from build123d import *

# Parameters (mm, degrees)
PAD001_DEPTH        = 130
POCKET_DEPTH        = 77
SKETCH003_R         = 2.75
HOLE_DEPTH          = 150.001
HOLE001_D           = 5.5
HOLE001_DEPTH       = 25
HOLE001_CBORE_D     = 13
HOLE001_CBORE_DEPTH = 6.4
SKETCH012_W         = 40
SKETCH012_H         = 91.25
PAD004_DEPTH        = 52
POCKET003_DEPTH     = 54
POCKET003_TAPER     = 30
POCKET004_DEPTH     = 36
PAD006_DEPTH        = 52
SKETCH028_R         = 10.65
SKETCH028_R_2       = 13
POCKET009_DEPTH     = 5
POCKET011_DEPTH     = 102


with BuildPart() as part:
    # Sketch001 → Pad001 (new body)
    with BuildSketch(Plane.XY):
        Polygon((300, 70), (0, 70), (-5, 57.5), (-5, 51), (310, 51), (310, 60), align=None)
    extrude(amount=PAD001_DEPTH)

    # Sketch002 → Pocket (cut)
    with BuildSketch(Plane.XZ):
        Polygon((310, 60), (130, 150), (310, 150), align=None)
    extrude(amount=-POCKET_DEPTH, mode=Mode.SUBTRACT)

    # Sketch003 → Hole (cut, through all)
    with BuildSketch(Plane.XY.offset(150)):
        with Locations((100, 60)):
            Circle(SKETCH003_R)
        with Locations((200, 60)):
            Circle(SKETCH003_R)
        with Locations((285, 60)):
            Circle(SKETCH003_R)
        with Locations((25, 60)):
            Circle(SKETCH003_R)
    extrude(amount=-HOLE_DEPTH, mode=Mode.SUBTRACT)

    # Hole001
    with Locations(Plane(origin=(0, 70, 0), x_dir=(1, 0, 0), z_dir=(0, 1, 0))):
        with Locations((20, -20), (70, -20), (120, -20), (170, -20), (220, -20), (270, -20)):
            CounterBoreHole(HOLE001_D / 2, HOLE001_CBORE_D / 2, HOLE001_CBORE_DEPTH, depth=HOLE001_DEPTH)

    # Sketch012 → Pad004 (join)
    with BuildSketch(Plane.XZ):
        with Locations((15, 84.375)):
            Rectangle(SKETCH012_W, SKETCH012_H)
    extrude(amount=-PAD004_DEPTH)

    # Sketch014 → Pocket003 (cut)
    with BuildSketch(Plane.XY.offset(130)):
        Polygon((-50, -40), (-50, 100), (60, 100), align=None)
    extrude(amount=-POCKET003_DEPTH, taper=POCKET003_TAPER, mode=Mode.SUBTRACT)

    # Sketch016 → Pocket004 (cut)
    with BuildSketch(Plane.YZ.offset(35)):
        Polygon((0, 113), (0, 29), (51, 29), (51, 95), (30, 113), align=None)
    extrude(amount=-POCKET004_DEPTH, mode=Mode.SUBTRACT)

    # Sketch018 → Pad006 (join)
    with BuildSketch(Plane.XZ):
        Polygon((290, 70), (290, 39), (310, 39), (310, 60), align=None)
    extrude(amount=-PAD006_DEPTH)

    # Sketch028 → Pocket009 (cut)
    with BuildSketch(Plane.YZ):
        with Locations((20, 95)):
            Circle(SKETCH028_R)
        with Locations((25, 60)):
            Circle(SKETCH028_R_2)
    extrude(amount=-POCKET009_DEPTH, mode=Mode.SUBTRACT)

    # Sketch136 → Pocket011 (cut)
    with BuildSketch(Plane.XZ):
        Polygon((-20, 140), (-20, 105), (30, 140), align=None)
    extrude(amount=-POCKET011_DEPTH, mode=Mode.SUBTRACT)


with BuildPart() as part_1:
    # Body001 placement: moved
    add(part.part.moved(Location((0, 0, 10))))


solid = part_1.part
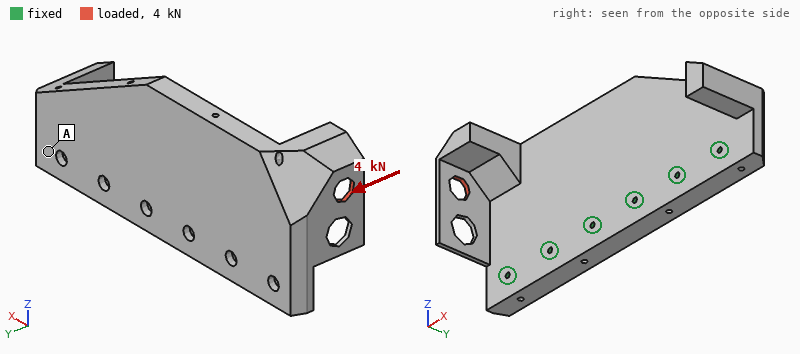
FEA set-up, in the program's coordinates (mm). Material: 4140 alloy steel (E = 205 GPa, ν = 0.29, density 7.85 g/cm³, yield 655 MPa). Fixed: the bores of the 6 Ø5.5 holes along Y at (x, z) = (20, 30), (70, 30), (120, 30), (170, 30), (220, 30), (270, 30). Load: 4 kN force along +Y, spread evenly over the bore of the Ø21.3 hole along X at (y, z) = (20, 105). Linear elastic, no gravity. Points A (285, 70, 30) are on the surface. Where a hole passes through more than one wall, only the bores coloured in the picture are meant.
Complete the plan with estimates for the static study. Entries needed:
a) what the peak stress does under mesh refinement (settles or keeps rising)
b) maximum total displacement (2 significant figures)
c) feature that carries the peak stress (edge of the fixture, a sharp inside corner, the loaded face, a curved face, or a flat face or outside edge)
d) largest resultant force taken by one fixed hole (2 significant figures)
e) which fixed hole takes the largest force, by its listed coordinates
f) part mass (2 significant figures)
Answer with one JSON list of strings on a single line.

["keeps rising", "0.18 mm", "edge of the fixture", "4.3 kN", "(20, 30)", "5.6 kg"]
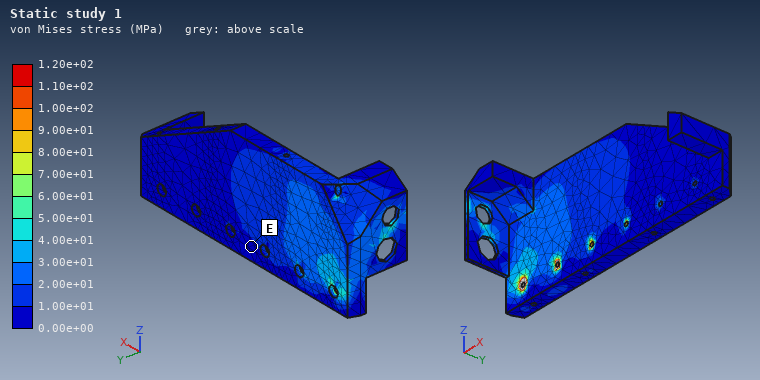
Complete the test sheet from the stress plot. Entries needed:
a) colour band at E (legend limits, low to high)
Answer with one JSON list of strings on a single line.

["0.00e+00 to 1.00e+01 MPa"]
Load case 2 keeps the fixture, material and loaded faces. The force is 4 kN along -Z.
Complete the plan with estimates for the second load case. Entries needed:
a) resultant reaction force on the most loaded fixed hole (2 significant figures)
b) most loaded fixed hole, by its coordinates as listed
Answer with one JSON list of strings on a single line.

["3.7 kN", "(20, 30)"]
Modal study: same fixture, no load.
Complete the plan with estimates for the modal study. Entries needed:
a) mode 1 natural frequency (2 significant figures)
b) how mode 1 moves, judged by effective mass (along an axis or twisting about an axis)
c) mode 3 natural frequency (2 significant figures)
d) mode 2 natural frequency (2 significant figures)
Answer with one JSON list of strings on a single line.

["860 Hz", "along Y", "1700 Hz", "1500 Hz"]
